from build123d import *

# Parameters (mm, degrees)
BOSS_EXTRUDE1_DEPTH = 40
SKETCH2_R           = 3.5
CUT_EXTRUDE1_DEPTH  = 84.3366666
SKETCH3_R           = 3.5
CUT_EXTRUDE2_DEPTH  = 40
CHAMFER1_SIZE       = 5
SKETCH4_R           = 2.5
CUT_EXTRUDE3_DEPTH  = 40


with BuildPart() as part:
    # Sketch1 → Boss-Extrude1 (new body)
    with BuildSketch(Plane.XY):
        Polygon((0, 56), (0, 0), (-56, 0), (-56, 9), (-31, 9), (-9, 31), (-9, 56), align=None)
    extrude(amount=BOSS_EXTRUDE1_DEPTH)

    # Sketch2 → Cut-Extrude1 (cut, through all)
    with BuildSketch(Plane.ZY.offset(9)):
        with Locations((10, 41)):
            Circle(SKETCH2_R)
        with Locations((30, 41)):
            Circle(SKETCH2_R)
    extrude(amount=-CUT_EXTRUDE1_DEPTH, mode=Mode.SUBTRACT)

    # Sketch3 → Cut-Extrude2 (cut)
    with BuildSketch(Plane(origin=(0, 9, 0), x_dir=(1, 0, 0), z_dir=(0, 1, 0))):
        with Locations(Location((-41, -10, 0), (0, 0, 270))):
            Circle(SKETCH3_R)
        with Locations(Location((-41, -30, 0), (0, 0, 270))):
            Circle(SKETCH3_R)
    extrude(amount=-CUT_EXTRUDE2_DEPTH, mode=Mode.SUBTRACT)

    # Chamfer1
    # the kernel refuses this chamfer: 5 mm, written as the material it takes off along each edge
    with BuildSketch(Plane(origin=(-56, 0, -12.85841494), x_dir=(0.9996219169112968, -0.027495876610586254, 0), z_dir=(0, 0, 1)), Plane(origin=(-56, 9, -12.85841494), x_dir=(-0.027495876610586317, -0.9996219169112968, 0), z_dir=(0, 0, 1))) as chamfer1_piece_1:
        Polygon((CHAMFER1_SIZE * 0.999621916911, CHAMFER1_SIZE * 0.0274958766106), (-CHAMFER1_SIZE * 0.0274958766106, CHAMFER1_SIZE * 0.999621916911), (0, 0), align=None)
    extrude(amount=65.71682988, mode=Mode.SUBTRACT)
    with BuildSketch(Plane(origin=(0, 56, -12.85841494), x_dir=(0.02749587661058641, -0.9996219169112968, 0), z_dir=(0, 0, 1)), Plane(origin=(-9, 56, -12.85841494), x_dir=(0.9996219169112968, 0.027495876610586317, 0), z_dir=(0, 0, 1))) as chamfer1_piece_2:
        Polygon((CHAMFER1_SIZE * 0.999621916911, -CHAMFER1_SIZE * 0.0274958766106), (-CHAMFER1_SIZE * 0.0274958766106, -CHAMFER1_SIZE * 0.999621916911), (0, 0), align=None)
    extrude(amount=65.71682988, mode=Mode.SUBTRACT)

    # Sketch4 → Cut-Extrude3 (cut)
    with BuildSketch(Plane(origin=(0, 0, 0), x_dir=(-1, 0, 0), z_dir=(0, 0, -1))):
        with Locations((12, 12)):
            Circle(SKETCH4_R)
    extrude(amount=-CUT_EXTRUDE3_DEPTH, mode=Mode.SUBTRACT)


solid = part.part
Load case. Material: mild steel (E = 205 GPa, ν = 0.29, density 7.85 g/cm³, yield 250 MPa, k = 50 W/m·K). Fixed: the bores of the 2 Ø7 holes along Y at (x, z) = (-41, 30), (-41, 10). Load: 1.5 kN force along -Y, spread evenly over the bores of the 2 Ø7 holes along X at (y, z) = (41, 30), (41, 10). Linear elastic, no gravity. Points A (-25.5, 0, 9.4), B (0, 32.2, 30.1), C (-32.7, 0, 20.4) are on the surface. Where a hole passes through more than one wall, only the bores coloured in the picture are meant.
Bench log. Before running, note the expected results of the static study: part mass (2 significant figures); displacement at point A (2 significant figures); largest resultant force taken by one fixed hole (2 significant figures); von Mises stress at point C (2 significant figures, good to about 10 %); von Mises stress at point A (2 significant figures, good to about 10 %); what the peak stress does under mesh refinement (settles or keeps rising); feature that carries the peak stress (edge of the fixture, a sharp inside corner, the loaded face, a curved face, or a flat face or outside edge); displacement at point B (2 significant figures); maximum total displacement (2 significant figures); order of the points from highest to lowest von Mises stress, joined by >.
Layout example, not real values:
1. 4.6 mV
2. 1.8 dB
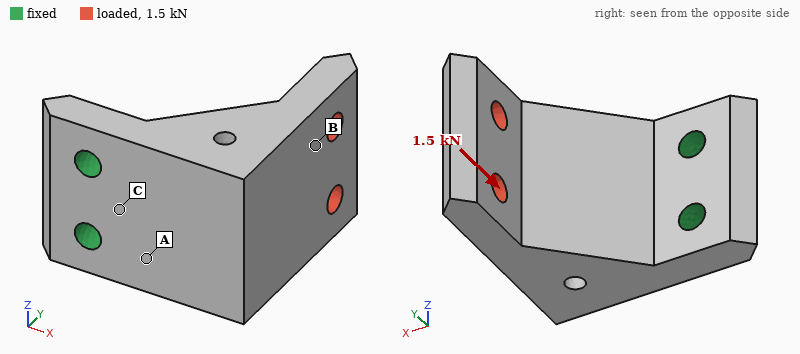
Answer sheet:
1. 330 g
2. 11 µm
3. 750 N
4. 61 MPa
5. 35 MPa
6. keeps rising
7. edge of the fixture
8. 53 µm
9. 72 µm
10. C > A > B
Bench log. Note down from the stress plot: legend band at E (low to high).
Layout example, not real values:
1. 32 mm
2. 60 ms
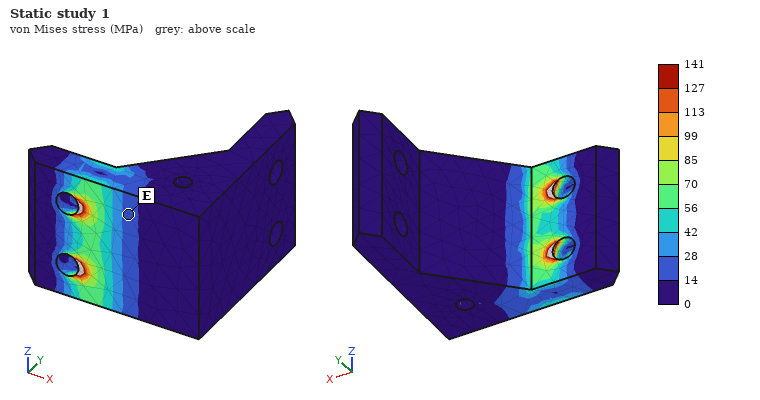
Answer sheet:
1. 14 to 28 MPa
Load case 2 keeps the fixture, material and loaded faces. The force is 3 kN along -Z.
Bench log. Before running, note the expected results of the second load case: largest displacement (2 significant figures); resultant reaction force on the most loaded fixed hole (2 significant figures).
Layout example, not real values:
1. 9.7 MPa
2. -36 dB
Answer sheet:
1. 63 µm
2. 6.0 kN
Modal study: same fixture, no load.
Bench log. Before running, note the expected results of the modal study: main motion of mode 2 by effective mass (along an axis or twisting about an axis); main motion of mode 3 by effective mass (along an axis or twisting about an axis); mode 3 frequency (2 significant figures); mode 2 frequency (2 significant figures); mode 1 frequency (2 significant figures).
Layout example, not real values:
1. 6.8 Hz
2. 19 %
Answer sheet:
1. along Z
2. along Z
3. 7900 Hz
4. 4000 Hz
5. 1800 Hz
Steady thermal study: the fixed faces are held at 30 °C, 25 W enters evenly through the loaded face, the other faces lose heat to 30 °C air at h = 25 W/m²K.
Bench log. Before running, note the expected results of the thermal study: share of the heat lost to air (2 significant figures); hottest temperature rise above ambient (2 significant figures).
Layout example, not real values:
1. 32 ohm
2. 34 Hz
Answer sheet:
1. 25 %
2. 55 K
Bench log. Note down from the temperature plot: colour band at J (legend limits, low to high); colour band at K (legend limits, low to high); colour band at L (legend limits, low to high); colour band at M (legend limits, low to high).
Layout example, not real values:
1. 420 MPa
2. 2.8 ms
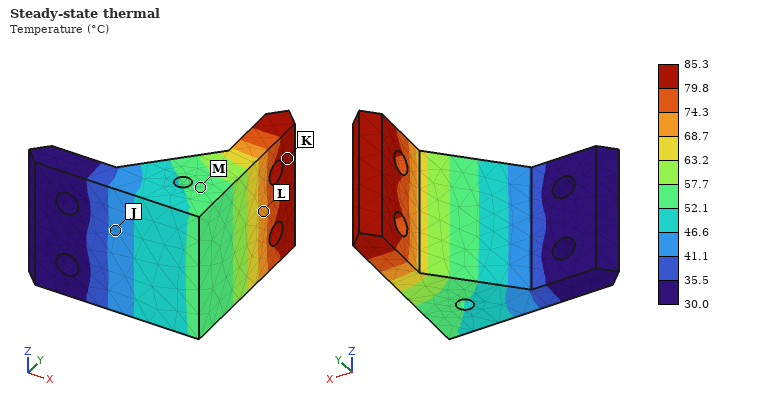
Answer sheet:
1. 41.1 to 46.6 °C
2. 79.8 to 85.3 °C
3. 68.7 to 74.3 °C
4. 52.1 to 57.7 °C
